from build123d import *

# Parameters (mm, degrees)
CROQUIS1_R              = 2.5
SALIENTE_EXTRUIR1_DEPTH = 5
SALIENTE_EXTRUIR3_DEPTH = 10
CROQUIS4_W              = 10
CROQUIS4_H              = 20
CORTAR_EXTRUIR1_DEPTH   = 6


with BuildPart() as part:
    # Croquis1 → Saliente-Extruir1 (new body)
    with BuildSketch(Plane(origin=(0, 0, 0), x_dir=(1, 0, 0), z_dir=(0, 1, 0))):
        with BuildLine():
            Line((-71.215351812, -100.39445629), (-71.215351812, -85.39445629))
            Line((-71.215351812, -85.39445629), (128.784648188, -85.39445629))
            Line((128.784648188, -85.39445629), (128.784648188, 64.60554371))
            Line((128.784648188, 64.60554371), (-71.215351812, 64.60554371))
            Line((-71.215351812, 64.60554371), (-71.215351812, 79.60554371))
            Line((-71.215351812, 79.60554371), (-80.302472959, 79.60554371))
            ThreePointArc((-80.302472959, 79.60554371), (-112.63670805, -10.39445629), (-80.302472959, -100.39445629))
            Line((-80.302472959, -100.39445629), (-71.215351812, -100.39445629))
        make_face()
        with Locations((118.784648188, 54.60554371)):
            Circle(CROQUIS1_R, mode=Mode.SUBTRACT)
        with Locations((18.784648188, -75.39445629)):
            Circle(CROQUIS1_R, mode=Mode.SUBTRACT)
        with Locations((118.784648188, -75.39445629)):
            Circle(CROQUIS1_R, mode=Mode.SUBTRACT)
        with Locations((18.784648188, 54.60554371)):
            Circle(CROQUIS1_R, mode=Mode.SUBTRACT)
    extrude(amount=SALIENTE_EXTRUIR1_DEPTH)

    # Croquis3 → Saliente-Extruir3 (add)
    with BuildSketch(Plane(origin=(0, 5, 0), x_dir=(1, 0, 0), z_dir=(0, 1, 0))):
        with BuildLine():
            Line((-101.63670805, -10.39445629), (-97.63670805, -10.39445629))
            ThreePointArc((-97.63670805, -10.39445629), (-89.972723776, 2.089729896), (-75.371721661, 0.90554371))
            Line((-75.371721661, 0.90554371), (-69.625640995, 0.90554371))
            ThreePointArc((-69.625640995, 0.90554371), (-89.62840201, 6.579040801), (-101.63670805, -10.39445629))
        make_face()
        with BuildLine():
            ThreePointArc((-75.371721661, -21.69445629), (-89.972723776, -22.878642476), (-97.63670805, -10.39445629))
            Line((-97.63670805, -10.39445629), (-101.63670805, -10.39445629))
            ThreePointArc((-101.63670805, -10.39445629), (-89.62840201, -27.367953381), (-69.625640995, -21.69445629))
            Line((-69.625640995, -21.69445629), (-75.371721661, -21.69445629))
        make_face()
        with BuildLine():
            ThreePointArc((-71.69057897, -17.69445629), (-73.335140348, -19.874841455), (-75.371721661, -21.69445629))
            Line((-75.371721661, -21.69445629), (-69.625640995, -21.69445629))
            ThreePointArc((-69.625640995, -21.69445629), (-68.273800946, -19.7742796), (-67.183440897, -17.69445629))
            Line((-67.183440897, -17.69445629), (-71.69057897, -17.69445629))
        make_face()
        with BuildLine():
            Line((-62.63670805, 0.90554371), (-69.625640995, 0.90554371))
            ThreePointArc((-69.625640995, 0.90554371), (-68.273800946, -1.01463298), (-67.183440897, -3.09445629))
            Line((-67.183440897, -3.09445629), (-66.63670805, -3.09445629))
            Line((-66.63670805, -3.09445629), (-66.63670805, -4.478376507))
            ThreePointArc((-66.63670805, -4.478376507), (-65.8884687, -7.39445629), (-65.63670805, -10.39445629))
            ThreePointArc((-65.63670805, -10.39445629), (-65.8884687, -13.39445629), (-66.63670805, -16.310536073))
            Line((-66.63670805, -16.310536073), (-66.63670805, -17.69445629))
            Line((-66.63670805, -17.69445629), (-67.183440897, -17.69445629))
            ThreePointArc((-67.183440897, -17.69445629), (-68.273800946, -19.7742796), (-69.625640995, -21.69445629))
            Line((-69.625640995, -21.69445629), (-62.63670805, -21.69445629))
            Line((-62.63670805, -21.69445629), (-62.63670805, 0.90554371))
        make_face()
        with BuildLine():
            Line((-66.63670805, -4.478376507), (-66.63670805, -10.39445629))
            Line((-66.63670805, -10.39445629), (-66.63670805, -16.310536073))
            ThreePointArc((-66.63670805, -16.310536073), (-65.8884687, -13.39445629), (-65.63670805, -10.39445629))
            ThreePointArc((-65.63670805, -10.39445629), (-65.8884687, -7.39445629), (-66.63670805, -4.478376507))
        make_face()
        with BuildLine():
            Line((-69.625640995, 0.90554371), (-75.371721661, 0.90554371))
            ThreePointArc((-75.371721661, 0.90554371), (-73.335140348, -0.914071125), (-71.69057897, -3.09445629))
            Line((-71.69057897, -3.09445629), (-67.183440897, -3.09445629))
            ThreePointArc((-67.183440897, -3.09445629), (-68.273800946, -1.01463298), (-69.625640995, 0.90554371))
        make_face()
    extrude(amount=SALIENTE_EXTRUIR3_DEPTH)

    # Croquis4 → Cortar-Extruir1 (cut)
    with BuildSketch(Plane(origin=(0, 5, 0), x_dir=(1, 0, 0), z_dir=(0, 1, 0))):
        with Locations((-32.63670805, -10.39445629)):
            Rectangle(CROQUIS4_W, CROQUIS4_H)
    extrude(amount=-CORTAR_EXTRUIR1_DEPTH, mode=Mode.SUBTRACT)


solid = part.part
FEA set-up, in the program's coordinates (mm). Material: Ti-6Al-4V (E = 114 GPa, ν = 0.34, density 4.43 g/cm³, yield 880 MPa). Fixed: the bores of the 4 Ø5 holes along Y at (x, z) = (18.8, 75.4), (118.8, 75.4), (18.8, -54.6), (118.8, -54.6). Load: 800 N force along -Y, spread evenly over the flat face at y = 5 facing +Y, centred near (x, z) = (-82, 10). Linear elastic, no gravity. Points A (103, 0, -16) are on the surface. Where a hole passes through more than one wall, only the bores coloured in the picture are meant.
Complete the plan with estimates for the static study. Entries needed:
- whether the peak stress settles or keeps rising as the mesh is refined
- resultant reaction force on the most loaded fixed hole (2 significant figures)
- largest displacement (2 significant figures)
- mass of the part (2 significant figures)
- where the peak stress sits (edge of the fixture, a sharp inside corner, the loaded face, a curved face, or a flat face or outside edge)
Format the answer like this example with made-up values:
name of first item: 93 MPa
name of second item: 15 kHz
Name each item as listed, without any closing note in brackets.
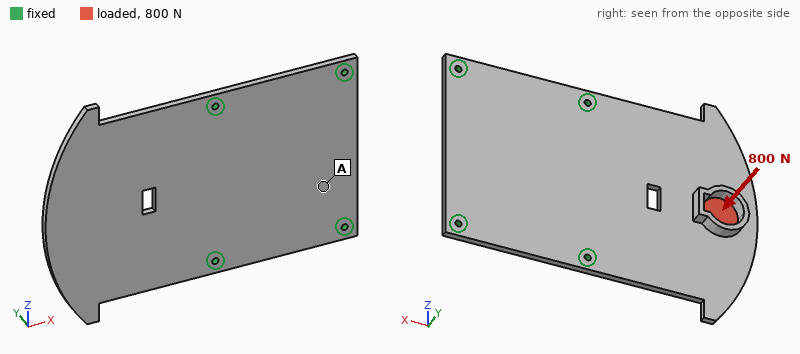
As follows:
whether the peak stress settles or keeps rising as the mesh is refined: keeps rising
resultant reaction force on the most loaded fixed hole: 580 N
largest displacement: 3.0 mm
mass of the part: 800 g
where the peak stress sits: edge of the fixture
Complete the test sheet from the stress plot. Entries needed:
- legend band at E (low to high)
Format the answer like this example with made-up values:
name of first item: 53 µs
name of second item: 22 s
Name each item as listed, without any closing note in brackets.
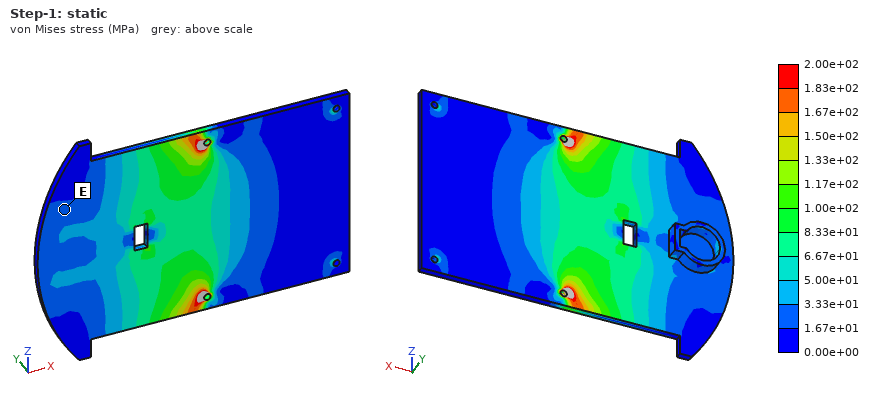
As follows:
legend band at E: 1.67e+01 to 3.33e+01 MPa
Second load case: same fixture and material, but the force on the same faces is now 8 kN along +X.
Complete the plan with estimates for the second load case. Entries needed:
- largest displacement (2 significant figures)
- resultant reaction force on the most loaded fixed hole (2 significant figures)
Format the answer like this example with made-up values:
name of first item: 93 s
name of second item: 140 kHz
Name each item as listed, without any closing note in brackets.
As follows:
largest displacement: 1.1 mm
resultant reaction force on the most loaded fixed hole: 3.2 kN
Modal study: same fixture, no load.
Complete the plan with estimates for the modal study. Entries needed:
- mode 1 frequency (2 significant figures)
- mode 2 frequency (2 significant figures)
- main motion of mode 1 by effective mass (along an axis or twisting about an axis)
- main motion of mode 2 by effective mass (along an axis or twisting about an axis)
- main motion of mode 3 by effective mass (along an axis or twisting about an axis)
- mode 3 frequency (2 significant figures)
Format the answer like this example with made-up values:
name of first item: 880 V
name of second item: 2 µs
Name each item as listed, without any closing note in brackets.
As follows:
mode 1 frequency: 210 Hz
mode 2 frequency: 570 Hz
main motion of mode 1 by effective mass: along Y
main motion of mode 2 by effective mass: twisting about X
main motion of mode 3 by effective mass: along Y
mode 3 frequency: 1200 Hz
